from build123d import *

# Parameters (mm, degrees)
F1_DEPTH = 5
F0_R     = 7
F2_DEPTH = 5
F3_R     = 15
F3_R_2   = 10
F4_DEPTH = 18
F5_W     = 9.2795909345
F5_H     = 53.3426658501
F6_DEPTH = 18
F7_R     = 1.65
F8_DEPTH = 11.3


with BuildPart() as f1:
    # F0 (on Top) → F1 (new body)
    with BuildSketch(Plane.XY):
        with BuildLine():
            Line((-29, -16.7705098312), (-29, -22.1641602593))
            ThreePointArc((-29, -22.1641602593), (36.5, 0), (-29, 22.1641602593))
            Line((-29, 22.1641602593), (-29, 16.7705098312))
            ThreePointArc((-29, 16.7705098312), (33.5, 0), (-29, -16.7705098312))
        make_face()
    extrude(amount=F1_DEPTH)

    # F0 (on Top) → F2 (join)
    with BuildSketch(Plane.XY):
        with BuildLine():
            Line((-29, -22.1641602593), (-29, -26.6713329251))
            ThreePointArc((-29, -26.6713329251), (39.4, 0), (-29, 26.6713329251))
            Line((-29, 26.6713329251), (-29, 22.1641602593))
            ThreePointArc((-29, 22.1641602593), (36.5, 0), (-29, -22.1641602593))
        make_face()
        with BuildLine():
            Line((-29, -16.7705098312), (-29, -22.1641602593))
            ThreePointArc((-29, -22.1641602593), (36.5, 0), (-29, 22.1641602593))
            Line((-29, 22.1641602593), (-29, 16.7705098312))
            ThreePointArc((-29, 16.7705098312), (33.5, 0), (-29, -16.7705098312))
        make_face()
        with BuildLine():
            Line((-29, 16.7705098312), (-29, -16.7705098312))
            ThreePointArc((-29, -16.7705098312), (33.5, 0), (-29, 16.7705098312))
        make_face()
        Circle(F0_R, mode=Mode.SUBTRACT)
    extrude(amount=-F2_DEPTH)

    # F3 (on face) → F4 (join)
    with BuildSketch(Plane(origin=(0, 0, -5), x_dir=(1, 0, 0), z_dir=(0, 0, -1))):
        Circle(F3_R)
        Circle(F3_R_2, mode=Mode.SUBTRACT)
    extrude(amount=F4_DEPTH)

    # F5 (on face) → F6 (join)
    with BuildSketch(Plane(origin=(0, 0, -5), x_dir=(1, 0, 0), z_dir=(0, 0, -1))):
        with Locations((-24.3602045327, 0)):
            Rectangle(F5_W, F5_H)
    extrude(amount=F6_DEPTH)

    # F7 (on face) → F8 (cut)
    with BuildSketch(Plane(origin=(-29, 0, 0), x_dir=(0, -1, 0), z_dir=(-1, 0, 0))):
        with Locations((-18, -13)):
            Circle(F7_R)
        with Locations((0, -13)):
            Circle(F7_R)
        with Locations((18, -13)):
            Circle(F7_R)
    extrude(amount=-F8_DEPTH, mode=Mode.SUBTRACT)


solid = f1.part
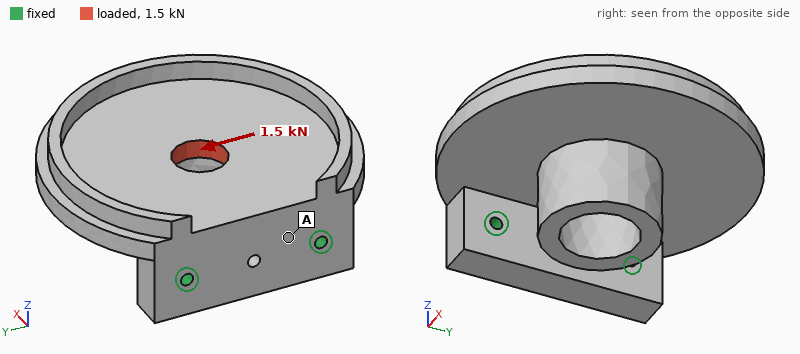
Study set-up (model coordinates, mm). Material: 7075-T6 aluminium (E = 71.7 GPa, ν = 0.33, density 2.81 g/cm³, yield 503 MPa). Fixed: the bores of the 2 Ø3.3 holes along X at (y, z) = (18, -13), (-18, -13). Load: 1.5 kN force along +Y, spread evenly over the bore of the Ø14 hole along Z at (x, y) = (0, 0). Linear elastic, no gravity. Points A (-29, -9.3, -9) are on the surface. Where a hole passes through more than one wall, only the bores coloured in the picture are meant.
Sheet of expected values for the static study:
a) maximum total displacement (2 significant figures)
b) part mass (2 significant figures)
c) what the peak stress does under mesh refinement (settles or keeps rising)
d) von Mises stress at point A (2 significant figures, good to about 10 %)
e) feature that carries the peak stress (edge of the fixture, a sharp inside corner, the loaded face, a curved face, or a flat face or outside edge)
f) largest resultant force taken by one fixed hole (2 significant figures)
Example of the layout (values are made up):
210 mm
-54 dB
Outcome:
31 µm
110 g
keeps rising
4.9 MPa
edge of the fixture
1.2 kN
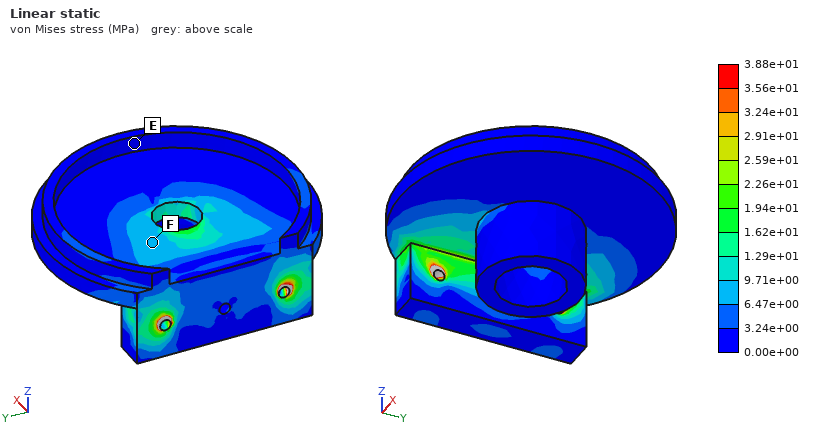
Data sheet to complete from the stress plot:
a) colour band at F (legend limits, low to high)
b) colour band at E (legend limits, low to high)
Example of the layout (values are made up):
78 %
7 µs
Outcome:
6.47e+00 to 9.71e+00 MPa
0.00e+00 to 3.24e+00 MPa
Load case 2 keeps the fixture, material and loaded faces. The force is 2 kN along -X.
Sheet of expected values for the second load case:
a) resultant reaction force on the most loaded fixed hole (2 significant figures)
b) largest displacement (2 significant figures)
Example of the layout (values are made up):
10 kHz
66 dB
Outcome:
1.0 kN
57 µm
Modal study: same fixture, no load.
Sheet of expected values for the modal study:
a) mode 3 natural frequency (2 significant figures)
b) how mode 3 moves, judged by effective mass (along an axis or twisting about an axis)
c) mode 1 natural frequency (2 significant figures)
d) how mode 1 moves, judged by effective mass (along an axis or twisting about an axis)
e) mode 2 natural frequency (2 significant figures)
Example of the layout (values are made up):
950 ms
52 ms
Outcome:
4200 Hz
along Y
1200 Hz
along Z
3200 Hz
